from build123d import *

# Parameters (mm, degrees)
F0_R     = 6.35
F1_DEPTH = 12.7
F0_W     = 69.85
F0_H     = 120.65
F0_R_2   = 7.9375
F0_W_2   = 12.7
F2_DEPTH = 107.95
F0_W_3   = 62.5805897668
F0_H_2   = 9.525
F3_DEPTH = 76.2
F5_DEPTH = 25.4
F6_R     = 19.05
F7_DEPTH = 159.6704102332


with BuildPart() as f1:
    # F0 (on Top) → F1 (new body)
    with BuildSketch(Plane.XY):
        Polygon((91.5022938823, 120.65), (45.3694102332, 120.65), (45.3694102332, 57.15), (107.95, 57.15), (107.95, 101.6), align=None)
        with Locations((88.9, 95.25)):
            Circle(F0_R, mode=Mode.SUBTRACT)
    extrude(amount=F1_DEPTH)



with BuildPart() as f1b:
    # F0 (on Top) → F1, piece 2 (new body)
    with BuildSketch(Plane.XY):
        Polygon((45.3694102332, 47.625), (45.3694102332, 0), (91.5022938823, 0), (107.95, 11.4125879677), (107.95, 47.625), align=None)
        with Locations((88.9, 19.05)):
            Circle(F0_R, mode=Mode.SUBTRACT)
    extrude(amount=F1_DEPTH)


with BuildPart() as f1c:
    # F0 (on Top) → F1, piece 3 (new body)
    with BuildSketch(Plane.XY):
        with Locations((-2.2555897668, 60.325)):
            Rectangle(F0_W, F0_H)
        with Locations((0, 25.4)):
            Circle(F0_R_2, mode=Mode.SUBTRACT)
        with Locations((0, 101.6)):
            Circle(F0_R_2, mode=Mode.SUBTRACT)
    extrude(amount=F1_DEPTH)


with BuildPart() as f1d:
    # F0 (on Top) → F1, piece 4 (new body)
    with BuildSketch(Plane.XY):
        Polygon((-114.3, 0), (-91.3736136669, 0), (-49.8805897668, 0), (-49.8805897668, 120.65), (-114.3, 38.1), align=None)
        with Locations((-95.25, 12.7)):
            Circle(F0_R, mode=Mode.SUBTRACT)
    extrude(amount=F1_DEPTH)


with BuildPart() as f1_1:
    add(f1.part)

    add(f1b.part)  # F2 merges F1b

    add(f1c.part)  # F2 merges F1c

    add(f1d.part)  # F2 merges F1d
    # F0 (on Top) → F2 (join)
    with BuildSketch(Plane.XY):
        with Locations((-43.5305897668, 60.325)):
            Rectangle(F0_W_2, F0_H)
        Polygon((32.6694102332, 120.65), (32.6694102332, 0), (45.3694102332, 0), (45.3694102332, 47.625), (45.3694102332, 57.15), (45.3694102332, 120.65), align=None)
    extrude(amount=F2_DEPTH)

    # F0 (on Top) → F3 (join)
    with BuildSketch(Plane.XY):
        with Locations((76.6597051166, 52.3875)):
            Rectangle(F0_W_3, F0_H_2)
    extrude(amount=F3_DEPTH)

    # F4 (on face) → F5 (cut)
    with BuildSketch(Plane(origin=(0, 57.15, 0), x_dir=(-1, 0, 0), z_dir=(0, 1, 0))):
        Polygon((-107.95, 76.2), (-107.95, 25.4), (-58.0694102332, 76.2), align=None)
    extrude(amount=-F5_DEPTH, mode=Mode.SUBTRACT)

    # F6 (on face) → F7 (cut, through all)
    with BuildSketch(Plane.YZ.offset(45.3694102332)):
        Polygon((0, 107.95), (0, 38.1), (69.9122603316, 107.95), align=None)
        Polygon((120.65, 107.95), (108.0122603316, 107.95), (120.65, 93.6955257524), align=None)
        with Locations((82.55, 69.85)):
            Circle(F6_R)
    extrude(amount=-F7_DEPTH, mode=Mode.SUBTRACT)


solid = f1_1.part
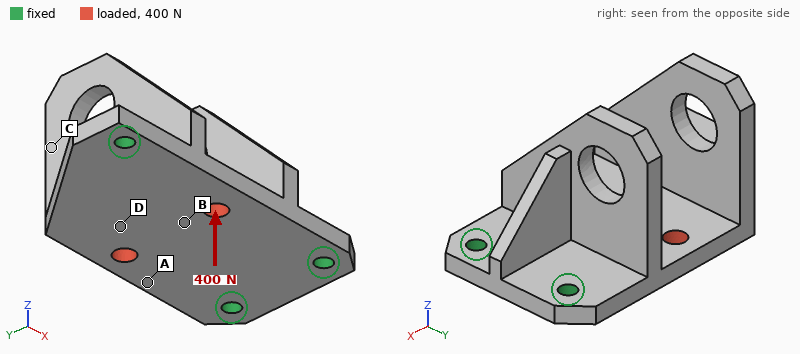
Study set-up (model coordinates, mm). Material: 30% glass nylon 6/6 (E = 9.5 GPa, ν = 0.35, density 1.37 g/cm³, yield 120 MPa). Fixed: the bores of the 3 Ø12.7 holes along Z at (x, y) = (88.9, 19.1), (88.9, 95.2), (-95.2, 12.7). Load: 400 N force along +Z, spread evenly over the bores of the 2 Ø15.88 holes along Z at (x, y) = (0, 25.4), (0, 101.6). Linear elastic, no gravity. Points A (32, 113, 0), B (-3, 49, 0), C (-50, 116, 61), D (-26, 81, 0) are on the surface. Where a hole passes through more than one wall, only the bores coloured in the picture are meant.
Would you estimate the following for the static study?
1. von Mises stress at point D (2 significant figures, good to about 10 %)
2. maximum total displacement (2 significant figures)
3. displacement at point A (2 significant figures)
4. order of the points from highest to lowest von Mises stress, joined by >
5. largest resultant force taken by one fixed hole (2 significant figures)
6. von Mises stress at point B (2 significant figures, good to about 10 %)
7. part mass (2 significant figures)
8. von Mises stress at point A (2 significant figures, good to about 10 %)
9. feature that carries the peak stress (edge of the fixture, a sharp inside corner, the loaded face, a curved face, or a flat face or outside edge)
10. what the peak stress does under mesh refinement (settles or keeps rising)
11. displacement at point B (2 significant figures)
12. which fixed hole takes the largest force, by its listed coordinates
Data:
1.7 MPa
0.18 mm
0.080 mm
B > D > A > C
190 N
2.5 MPa
710 g
1.00 MPa
edge of the fixture
keeps rising
0.088 mm
(88.9, 95.2)
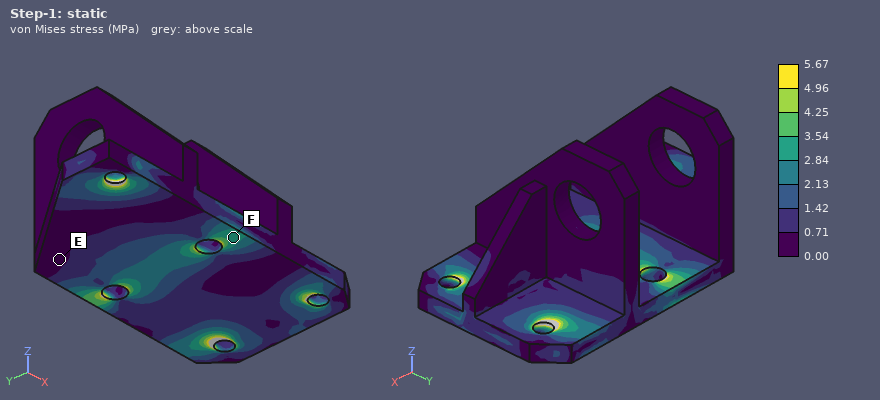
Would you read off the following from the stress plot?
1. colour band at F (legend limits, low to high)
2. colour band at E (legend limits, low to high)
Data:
2.84 to 3.54 MPa
0.00 to 0.71 MPa
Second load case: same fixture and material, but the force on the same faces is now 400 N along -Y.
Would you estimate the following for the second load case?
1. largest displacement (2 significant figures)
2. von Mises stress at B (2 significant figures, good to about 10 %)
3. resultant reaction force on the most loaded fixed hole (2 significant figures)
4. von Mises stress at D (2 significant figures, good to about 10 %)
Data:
6.3 µm
0.16 MPa
190 N
0.28 MPa
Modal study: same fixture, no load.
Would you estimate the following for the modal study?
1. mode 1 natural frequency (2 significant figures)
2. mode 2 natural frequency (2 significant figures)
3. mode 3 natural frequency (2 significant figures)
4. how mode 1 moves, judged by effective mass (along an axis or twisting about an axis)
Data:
400 Hz
520 Hz
790 Hz
along Z
